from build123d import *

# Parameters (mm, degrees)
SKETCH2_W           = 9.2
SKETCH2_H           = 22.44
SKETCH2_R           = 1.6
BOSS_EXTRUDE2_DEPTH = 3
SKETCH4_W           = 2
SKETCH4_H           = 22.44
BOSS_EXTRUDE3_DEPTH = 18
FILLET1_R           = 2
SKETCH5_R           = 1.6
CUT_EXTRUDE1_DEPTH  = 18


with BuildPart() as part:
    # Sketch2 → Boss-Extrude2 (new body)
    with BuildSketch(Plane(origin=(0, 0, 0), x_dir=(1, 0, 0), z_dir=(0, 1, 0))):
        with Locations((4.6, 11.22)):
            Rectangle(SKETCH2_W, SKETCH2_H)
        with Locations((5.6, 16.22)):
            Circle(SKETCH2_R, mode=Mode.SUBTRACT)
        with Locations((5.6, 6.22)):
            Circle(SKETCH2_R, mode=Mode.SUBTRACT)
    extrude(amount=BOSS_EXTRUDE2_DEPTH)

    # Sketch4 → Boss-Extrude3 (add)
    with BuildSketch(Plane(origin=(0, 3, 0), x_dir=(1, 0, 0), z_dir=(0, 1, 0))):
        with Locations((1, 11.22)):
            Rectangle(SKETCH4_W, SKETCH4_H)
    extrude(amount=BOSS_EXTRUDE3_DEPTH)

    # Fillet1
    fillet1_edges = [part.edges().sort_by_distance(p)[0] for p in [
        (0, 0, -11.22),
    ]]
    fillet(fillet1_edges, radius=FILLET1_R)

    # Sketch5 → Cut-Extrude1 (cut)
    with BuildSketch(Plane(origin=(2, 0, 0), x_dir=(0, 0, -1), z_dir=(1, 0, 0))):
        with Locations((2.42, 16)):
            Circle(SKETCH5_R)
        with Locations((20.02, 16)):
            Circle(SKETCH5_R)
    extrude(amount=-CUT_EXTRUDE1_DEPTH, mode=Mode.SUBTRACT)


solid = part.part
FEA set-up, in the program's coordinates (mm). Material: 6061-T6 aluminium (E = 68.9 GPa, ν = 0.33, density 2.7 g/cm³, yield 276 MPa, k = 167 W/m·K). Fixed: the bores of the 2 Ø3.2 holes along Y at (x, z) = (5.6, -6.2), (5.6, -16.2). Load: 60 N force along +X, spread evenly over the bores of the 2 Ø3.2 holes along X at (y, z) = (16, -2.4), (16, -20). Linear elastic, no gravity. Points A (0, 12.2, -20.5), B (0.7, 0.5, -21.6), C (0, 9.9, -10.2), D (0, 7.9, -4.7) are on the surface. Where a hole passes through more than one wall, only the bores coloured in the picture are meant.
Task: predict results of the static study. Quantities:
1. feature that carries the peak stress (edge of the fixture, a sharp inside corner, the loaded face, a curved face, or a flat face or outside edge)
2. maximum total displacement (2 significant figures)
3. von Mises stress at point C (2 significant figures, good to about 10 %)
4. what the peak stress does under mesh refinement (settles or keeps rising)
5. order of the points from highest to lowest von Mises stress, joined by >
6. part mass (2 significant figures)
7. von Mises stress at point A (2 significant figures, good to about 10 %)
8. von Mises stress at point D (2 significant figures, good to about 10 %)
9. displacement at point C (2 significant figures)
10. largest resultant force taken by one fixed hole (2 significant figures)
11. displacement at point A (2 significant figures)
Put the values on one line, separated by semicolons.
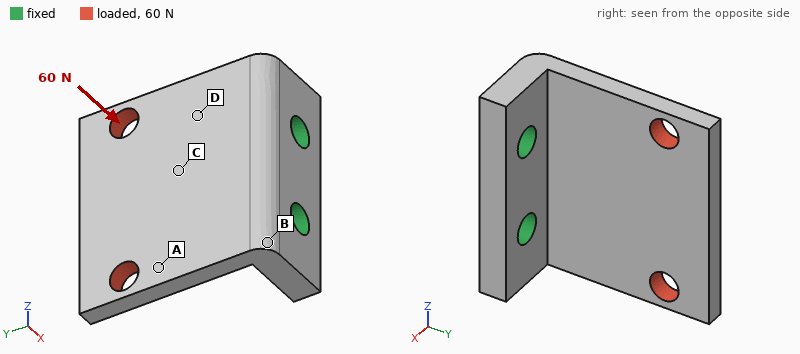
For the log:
edge of the fixture; 95 µm; 21 MPa; keeps rising; D > C > A > B; 3.6 g; 16 MPa; 29 MPa; 27 µm; 30 N; 40 µm
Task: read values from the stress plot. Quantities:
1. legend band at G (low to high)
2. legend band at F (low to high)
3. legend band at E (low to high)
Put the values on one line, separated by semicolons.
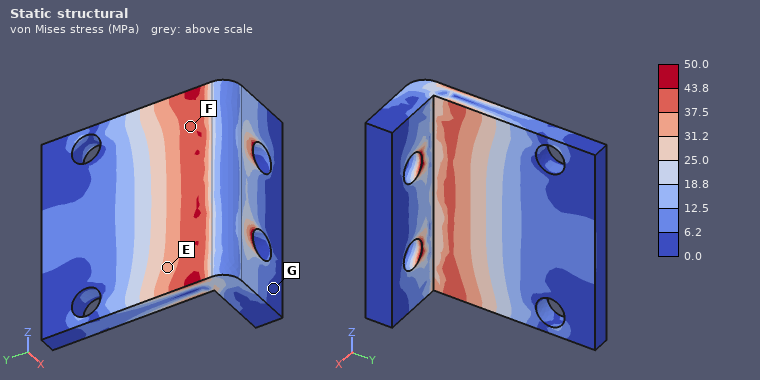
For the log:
0.0 to 6.2 MPa; 37.5 to 43.8 MPa; 31.2 to 37.5 MPa
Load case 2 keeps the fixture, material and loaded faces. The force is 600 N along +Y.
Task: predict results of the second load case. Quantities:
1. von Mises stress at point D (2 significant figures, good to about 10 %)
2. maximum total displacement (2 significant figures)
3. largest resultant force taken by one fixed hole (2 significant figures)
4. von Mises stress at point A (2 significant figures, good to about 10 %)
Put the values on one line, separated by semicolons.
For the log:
15 MPa; 35 µm; 300 N; 20 MPa
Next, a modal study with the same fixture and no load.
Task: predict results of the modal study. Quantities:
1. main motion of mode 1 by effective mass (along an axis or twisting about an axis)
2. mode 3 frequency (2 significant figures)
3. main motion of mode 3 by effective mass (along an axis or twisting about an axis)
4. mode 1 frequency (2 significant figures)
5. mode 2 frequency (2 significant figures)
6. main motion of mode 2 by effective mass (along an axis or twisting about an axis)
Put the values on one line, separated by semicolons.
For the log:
along X; 15 kHz; along Z; 4300 Hz; 9300 Hz; twisting about Y
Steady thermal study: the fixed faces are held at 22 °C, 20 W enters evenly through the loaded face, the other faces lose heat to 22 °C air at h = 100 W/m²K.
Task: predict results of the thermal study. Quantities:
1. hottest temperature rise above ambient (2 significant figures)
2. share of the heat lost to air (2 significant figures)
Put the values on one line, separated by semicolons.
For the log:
50 K; 14 %
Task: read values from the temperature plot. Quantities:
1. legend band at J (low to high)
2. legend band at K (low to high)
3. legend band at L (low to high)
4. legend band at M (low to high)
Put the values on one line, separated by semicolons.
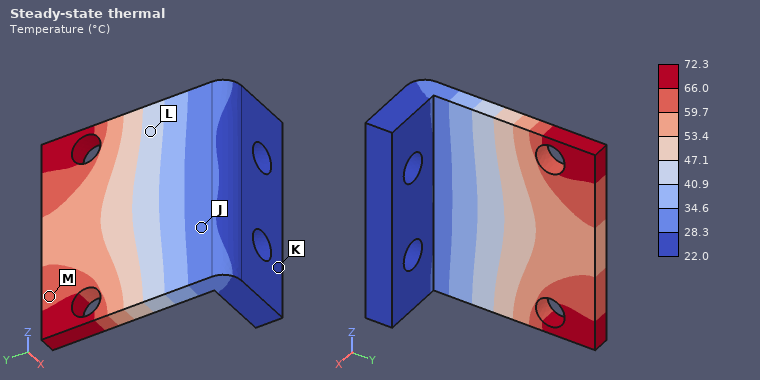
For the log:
28.3 to 34.6 °C; 22.0 to 28.3 °C; 40.9 to 47.1 °C; 59.7 to 66.0 °C
